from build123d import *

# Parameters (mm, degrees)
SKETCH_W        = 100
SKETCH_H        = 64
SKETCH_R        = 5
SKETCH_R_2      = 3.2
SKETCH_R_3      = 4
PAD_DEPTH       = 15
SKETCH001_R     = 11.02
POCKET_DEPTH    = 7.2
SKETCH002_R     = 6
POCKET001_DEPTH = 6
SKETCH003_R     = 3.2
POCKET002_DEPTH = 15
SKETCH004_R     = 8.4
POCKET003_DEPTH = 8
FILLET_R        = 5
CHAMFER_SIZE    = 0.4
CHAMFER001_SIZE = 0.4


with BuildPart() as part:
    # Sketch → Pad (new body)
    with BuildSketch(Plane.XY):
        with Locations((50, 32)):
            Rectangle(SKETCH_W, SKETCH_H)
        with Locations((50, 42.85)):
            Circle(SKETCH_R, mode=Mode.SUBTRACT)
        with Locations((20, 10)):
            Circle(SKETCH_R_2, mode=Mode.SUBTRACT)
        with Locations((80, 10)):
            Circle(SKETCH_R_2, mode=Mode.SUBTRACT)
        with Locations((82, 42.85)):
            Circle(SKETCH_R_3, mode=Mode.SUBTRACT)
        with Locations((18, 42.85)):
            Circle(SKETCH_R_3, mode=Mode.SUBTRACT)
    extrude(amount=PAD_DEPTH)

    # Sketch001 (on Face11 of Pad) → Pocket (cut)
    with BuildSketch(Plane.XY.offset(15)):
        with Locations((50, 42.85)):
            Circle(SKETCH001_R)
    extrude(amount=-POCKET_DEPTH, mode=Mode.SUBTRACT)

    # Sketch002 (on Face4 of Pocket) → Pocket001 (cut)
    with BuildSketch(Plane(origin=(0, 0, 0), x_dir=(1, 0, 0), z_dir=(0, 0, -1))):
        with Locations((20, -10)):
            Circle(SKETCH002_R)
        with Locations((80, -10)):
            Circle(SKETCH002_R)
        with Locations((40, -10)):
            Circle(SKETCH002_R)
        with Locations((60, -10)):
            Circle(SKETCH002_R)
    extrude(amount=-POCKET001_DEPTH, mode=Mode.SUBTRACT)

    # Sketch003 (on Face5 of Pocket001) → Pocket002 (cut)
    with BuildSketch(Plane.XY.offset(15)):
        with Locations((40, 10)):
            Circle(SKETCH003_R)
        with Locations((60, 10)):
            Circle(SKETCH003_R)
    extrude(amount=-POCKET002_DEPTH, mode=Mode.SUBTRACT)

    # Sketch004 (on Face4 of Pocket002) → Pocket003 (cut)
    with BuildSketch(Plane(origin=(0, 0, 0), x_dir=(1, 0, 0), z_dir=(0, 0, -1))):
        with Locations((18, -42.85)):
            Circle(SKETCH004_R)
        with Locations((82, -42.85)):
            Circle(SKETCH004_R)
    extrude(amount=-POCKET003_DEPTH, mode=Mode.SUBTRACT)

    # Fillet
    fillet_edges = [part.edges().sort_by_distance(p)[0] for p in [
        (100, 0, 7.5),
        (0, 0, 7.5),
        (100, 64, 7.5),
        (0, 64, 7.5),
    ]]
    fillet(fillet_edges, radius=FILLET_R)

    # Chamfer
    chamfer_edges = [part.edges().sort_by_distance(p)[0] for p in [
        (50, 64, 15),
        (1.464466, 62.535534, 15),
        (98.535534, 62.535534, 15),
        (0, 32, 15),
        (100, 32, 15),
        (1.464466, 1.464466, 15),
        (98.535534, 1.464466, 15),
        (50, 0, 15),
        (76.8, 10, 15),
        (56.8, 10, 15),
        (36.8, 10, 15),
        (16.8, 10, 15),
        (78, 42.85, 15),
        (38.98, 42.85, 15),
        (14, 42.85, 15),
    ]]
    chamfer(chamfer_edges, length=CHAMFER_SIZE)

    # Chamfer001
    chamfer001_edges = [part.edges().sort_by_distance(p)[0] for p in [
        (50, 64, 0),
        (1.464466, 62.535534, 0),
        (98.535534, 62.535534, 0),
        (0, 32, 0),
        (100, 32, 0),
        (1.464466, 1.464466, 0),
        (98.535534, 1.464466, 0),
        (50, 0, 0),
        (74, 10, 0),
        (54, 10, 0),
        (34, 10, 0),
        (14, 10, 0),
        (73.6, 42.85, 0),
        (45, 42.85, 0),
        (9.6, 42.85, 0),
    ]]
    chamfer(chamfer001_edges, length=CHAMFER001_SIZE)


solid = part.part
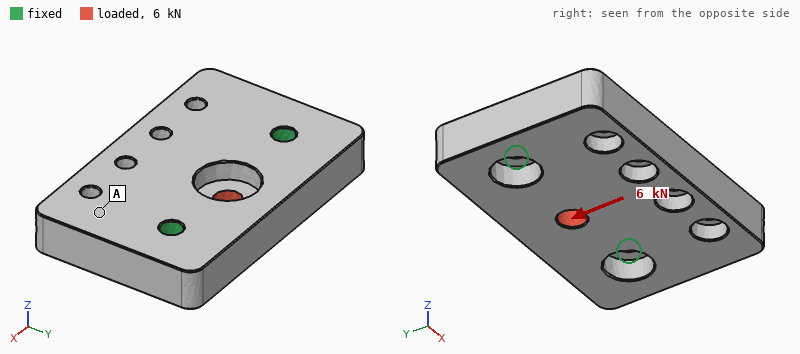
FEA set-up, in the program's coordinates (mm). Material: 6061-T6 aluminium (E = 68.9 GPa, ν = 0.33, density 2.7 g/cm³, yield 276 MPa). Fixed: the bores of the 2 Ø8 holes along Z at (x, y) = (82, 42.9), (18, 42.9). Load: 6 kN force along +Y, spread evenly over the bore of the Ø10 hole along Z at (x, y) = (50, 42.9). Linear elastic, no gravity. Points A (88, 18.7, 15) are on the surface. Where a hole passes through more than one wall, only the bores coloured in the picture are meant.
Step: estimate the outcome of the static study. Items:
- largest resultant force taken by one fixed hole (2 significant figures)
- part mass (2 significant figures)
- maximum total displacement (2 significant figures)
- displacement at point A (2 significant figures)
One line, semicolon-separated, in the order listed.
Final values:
3.0 kN; 230 g; 52 µm; 24 µm
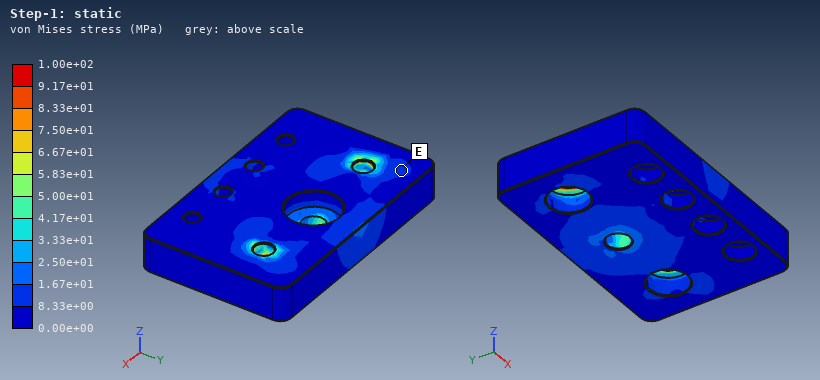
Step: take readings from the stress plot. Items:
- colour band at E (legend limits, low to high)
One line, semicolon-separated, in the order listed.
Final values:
8.33e+00 to 1.67e+01 MPa
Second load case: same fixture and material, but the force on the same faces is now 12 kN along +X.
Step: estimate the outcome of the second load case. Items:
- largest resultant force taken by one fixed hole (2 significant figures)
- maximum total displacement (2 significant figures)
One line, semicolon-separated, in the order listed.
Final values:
6.1 kN; 16 µm
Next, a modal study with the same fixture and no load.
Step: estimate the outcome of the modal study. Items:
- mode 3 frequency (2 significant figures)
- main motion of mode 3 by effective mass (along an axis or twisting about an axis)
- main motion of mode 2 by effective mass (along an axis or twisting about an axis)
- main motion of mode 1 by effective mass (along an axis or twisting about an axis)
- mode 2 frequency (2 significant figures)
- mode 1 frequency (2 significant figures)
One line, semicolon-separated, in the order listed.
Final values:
8400 Hz; along Z; twisting about Y; along Z; 5700 Hz; 2900 Hz
